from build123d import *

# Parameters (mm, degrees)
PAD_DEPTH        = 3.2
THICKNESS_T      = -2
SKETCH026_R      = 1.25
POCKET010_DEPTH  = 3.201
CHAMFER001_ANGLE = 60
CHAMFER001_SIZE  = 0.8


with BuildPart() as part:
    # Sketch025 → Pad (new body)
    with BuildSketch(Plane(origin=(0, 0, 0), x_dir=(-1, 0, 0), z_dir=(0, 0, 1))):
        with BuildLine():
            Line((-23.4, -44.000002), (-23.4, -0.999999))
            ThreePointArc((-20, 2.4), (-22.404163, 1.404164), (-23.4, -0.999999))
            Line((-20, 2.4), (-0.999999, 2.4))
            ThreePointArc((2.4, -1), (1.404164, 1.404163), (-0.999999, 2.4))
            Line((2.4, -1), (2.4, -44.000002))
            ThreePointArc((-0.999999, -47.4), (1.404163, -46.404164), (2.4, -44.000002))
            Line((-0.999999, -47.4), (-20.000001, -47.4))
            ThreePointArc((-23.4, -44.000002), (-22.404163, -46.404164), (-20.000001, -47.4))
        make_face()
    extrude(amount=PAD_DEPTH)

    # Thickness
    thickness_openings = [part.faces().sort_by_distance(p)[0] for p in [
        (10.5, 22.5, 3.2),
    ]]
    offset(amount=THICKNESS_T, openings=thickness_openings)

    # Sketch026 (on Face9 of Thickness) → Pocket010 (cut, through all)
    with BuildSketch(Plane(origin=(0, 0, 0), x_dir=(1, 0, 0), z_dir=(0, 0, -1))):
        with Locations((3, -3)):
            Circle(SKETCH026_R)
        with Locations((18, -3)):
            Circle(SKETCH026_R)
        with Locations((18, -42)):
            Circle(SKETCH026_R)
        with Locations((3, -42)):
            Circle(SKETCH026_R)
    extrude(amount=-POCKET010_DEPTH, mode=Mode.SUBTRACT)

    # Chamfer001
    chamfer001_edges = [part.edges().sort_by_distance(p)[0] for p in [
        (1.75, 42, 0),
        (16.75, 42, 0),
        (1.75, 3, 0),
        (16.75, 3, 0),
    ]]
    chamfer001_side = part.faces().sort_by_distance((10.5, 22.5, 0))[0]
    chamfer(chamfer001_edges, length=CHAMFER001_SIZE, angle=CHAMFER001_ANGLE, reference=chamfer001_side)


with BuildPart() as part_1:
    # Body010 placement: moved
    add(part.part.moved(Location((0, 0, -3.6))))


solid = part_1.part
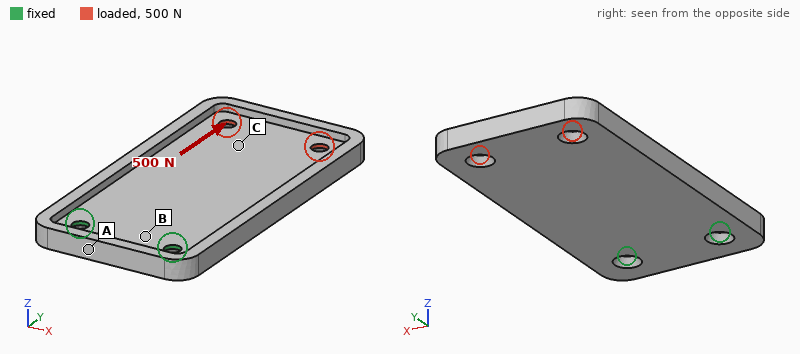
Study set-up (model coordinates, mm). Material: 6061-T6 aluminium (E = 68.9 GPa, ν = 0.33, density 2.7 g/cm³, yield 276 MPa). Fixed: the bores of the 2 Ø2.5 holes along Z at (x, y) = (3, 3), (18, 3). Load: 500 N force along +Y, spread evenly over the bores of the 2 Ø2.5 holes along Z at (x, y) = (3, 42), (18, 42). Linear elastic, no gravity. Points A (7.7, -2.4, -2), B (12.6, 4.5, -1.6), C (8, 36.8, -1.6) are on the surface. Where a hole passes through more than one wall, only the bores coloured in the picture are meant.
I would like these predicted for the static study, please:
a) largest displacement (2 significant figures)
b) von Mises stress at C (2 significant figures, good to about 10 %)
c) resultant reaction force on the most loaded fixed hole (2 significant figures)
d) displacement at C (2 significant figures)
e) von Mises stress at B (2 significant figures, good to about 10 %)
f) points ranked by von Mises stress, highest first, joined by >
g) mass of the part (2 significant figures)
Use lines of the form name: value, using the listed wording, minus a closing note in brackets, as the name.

largest displacement: 0.14 mm
von Mises stress at C: 18 MPa
resultant reaction force on the most loaded fixed hole: 250 N
displacement at C: 0.079 mm
von Mises stress at B: 12 MPa
points ranked by von Mises stress, highest first, joined by >: C > B > A
mass of the part: 7.6 g
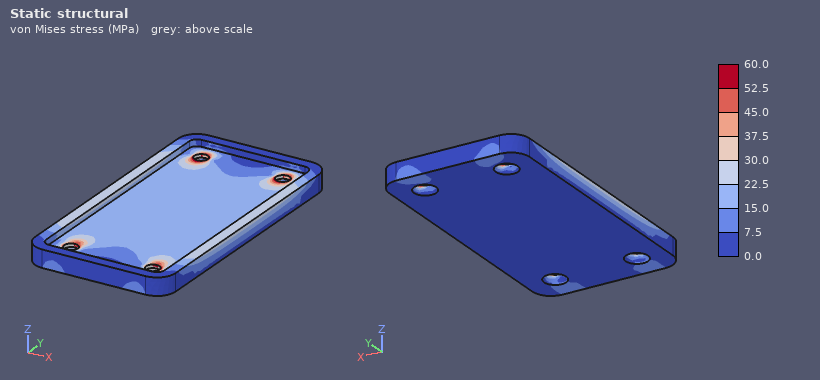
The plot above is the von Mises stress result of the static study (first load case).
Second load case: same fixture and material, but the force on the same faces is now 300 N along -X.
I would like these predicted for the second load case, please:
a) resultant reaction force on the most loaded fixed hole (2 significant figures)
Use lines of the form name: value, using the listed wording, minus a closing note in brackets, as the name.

resultant reaction force on the most loaded fixed hole: 740 N
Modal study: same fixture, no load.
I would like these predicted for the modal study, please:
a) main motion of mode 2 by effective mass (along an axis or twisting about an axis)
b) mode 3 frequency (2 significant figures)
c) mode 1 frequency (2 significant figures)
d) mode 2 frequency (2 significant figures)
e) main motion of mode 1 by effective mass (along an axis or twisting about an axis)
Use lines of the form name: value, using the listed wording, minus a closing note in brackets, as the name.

main motion of mode 2 by effective mass: twisting about Y
mode 3 frequency: 5200 Hz
mode 1 frequency: 790 Hz
mode 2 frequency: 2900 Hz
main motion of mode 1 by effective mass: along Z
